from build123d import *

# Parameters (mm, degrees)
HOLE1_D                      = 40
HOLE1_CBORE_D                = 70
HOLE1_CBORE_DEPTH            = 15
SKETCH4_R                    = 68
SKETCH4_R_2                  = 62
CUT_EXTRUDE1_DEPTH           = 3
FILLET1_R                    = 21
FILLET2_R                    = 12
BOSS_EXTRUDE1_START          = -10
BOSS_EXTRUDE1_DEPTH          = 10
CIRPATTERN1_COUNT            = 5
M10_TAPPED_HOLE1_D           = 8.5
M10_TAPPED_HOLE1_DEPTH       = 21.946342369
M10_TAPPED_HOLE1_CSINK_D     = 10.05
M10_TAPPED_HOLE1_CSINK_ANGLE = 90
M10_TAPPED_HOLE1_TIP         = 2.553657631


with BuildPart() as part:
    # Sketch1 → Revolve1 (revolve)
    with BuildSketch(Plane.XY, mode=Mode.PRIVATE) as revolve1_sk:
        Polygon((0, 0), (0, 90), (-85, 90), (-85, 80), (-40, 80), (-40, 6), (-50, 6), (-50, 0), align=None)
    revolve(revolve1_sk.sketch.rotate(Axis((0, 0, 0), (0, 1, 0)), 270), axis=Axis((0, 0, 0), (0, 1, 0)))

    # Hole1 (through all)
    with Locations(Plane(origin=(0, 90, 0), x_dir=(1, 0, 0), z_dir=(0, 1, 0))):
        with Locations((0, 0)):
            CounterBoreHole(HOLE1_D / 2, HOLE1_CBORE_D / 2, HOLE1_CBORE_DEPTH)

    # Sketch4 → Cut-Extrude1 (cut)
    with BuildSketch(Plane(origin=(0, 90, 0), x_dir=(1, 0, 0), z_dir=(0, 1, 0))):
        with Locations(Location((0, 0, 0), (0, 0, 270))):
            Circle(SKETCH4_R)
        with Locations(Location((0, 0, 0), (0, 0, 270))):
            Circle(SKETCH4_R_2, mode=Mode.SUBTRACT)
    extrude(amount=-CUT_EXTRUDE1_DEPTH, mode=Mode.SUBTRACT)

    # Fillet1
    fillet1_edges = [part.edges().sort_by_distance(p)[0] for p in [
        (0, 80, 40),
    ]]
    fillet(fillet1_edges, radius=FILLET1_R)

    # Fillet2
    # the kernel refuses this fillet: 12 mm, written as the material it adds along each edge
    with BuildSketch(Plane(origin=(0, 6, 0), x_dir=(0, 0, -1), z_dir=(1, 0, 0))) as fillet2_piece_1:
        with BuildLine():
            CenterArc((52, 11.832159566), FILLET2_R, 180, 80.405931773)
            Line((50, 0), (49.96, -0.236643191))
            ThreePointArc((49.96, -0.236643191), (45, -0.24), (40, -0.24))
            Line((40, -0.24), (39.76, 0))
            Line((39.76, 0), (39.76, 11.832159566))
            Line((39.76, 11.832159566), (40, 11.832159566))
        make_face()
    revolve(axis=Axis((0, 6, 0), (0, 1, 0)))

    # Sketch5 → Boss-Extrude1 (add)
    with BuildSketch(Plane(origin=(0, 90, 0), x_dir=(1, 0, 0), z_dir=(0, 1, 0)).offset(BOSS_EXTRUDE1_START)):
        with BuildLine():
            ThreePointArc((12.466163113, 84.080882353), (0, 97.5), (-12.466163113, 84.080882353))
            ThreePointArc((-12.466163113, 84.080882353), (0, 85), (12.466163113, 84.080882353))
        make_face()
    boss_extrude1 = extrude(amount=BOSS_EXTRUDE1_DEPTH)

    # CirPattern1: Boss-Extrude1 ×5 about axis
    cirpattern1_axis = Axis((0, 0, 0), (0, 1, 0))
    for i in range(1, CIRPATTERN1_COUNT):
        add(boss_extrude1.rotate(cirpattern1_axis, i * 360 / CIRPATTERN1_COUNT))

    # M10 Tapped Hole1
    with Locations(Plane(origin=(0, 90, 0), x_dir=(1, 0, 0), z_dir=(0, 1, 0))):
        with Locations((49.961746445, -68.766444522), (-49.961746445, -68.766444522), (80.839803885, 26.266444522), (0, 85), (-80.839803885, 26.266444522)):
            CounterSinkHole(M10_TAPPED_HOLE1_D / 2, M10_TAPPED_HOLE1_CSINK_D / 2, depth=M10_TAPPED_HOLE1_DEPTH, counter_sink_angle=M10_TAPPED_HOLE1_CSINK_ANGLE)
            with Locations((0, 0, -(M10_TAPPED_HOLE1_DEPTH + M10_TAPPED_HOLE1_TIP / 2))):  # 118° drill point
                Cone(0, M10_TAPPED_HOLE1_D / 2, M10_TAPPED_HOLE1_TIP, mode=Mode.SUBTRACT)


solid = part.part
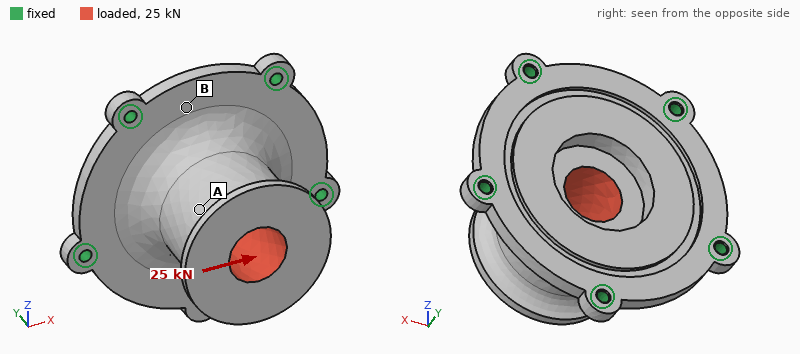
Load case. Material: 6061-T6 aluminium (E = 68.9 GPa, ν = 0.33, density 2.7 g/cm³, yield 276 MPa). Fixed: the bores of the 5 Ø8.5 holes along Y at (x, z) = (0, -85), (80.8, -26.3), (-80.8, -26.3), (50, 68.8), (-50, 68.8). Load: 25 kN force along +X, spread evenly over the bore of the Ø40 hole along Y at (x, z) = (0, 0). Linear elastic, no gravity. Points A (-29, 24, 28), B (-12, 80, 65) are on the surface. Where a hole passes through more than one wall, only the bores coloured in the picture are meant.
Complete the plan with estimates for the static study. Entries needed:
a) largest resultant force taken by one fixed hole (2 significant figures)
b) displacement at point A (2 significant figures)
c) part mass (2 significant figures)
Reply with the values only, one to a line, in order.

10 kN
0.18 mm
1.4 kg
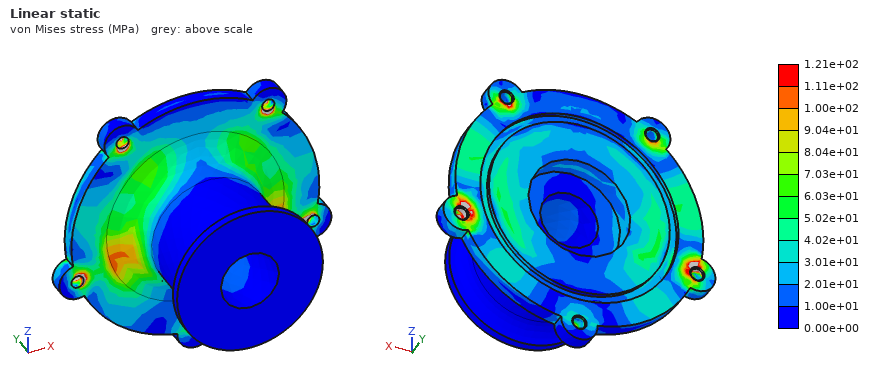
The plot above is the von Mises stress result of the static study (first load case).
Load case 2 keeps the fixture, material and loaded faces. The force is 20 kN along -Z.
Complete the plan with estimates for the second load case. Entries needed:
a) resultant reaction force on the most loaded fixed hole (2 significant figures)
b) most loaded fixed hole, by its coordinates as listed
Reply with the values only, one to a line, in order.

8.4 kN
(0, -85)
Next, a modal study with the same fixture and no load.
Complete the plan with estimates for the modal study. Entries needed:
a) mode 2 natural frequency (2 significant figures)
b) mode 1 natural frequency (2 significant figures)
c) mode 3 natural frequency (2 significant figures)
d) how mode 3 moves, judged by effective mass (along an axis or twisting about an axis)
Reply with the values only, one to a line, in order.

1900 Hz
1800 Hz
2100 Hz
along Y
